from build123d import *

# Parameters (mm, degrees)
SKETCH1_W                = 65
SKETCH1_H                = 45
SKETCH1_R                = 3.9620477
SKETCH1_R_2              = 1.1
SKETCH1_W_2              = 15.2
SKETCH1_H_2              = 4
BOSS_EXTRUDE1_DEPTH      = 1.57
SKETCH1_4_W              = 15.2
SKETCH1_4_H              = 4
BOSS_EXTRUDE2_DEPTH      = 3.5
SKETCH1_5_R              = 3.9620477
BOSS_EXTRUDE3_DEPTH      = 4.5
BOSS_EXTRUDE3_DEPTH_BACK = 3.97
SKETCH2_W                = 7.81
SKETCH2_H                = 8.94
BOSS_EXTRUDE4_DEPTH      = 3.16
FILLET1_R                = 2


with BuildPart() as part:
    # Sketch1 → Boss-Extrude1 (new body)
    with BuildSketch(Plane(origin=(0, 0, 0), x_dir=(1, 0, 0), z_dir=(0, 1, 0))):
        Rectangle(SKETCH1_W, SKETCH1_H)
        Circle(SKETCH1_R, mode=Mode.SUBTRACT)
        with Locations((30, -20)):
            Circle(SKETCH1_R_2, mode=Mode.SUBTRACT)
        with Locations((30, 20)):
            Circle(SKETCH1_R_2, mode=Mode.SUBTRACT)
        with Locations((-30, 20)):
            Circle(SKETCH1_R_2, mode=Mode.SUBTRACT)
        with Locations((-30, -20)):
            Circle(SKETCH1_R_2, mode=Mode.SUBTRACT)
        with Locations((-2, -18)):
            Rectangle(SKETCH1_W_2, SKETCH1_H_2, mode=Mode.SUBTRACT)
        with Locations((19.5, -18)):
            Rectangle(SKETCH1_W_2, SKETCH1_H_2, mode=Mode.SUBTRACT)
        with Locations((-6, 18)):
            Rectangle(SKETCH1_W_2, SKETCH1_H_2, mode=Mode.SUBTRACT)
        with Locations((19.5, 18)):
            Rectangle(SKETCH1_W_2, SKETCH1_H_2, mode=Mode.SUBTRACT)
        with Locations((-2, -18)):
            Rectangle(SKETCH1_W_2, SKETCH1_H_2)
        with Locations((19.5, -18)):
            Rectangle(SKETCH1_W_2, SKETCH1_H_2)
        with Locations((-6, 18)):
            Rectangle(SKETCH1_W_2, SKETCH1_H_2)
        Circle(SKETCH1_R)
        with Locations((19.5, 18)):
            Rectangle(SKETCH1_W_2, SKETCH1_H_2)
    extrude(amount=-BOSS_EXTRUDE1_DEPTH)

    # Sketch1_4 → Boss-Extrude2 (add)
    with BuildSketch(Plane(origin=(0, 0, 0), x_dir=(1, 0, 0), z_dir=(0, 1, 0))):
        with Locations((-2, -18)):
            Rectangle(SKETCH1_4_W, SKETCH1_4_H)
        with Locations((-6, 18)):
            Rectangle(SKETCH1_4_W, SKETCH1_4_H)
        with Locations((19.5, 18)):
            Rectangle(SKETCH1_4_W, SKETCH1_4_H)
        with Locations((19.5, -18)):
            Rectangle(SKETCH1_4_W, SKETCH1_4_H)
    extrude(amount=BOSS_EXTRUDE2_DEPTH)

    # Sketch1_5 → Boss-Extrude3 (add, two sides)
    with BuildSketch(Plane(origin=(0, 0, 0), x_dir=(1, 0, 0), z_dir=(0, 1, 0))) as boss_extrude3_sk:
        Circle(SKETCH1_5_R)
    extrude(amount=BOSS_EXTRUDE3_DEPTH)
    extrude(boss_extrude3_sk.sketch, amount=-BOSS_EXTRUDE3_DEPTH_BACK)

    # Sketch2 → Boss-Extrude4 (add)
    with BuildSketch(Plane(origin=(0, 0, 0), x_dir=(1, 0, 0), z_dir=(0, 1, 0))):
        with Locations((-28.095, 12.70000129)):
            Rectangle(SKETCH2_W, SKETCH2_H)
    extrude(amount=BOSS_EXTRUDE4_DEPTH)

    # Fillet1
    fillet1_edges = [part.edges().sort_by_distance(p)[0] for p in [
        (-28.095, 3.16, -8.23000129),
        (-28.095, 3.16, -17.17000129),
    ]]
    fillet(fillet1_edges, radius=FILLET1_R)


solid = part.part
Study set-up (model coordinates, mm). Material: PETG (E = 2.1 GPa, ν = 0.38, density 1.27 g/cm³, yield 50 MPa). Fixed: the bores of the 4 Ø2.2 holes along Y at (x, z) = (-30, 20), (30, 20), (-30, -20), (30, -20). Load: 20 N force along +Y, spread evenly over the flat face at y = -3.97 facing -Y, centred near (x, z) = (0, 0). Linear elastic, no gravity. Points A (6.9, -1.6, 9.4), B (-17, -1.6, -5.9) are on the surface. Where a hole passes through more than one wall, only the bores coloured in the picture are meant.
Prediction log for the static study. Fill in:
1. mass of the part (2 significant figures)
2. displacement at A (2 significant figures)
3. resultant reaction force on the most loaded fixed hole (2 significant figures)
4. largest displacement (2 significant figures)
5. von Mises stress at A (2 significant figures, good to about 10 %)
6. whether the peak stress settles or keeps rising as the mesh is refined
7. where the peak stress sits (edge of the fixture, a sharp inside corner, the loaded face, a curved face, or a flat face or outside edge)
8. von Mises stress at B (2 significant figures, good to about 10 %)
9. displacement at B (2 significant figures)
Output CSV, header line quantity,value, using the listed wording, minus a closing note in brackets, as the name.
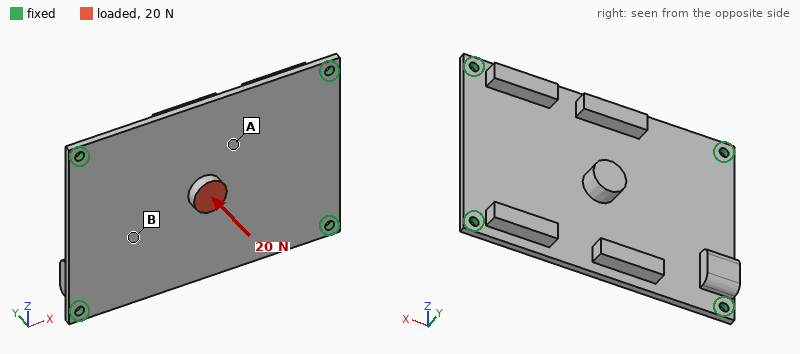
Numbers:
quantity,value
mass of the part,7.6 g
displacement at A,0.68 mm
resultant reaction force on the most loaded fixed hole,5.2 N
largest displacement,0.80 mm
von Mises stress at A,5.5 MPa
whether the peak stress settles or keeps rising as the mesh is refined,keeps rising
where the peak stress sits,edge of the fixture
von Mises stress at B,2.0 MPa
displacement at B,0.44 mm
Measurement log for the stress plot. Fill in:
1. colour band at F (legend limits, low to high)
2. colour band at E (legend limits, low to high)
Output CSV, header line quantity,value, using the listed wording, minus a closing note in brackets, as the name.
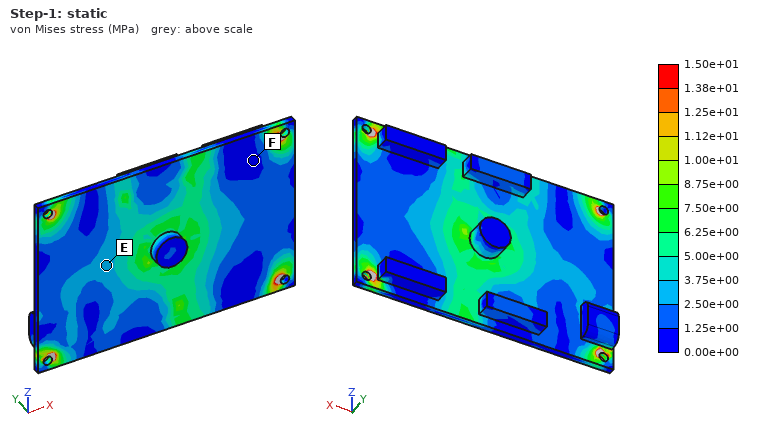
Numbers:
quantity,value
colour band at F,0.00e+00 to 1.25e+00 MPa
colour band at E,2.50e+00 to 3.75e+00 MPa
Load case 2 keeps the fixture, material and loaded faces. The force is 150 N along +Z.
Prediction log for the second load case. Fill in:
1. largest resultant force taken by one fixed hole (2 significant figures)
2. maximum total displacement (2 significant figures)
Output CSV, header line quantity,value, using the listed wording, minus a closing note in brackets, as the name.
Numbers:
quantity,value
largest resultant force taken by one fixed hole,48 N
maximum total displacement,0.72 mm
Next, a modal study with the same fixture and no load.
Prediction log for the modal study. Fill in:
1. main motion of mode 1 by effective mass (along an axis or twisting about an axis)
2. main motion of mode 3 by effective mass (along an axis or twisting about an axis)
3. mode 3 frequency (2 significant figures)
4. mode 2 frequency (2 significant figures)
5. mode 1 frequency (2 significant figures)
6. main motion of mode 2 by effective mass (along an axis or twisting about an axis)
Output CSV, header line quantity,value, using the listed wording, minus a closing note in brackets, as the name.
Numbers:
quantity,value
main motion of mode 1 by effective mass,along Y
main motion of mode 3 by effective mass,twisting about Z
mode 3 frequency,1200 Hz
mode 2 frequency,780 Hz
mode 1 frequency,470 Hz
main motion of mode 2 by effective mass,twisting about X
